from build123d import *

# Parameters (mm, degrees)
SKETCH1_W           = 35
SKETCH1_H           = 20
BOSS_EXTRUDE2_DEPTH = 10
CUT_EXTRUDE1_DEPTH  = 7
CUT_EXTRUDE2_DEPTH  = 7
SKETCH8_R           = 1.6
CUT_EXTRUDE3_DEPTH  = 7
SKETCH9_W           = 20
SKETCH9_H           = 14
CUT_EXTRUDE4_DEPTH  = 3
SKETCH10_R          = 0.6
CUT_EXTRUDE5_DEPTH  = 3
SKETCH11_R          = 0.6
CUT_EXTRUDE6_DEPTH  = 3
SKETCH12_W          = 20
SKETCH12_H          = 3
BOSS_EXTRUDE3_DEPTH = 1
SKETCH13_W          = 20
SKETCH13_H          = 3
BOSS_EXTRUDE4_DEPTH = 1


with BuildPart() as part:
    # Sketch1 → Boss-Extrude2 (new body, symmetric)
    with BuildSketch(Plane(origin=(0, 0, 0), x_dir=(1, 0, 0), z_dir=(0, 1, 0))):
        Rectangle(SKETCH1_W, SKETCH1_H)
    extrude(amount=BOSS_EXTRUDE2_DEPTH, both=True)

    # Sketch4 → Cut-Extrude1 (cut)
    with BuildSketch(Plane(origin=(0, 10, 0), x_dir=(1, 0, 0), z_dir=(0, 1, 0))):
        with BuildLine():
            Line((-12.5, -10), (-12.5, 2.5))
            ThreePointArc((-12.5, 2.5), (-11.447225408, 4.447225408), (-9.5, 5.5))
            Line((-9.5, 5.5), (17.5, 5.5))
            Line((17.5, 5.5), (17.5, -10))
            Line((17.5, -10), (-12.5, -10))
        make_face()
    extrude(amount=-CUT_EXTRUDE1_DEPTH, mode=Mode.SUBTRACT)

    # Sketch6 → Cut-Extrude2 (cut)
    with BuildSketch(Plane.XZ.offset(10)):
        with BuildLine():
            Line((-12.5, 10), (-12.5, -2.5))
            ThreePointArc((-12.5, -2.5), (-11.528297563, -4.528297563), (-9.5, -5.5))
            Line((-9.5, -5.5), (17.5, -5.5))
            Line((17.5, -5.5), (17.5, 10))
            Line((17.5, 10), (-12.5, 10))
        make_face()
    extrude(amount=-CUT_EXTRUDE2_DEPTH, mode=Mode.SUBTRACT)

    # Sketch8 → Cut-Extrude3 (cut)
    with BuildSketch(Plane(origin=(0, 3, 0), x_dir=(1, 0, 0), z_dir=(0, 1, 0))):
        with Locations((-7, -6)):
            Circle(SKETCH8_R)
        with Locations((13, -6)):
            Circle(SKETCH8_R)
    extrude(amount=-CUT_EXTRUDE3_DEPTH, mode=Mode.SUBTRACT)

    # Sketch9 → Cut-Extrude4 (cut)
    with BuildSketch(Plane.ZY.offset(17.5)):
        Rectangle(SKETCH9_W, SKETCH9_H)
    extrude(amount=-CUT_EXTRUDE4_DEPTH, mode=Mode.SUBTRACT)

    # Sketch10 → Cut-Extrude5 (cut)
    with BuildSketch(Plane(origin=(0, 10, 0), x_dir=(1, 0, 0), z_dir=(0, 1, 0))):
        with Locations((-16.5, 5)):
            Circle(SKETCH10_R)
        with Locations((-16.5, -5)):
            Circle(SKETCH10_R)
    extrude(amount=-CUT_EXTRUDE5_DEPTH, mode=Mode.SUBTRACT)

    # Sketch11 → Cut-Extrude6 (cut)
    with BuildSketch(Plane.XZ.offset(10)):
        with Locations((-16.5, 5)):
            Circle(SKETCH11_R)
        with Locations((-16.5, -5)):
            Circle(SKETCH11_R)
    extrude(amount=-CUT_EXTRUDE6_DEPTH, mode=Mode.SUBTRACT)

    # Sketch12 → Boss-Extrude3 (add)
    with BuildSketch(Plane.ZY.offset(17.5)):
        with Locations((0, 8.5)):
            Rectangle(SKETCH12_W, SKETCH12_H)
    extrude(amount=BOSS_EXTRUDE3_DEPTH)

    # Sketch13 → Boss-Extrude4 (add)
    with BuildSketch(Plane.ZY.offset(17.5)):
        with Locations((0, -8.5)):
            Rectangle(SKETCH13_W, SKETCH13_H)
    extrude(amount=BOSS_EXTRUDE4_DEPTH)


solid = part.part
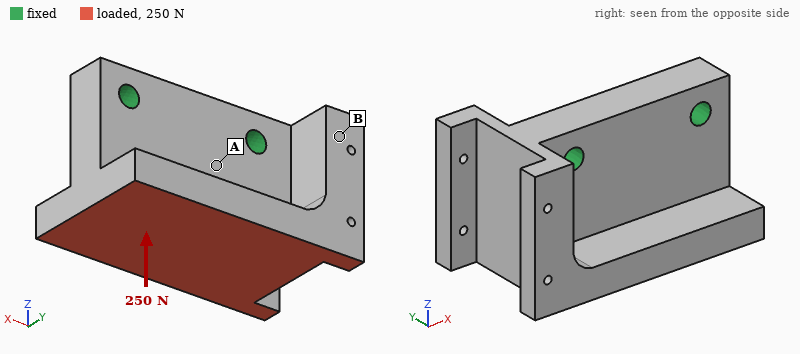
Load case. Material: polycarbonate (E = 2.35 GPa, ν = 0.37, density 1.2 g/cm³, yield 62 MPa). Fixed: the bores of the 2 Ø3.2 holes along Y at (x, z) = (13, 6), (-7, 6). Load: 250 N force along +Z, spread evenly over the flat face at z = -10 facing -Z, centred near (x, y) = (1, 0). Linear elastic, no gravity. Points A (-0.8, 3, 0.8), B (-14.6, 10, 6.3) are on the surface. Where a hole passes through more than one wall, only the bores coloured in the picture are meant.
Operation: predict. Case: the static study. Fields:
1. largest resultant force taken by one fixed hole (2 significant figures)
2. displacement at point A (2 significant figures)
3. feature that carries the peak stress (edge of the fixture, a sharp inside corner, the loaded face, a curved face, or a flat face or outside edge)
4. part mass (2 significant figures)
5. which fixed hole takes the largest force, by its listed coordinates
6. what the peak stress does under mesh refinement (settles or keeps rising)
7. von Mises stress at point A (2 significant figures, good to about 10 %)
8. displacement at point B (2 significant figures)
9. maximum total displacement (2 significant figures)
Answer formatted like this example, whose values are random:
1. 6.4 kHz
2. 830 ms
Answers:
1. 150 N
2. 6.7 µm
3. edge of the fixture
4. 8.0 g
5. (-7, 6)
6. keeps rising
7. 1.2 MPa
8. 12 µm
9. 26 µm
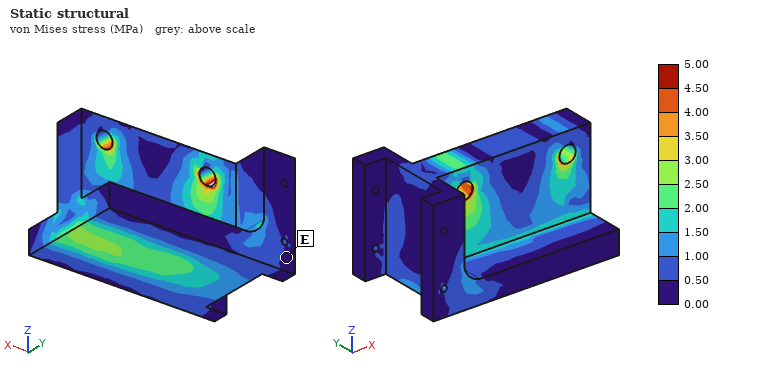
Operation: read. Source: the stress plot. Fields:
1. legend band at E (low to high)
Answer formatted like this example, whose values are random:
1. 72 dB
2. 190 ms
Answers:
1. 0.00 to 0.50 MPa
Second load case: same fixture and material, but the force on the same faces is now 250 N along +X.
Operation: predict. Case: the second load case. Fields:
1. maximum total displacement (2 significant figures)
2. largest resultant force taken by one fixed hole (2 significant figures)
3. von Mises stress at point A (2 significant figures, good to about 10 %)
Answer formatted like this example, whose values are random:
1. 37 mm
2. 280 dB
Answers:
1. 61 µm
2. 220 N
3. 3.4 MPa
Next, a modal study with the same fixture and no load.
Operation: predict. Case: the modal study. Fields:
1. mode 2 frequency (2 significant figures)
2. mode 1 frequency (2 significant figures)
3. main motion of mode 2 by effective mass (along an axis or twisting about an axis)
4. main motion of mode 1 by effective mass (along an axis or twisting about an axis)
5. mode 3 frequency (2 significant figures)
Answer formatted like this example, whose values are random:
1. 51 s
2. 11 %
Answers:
1. 3400 Hz
2. 2400 Hz
3. twisting about Z
4. along Y
5. 5600 Hz
